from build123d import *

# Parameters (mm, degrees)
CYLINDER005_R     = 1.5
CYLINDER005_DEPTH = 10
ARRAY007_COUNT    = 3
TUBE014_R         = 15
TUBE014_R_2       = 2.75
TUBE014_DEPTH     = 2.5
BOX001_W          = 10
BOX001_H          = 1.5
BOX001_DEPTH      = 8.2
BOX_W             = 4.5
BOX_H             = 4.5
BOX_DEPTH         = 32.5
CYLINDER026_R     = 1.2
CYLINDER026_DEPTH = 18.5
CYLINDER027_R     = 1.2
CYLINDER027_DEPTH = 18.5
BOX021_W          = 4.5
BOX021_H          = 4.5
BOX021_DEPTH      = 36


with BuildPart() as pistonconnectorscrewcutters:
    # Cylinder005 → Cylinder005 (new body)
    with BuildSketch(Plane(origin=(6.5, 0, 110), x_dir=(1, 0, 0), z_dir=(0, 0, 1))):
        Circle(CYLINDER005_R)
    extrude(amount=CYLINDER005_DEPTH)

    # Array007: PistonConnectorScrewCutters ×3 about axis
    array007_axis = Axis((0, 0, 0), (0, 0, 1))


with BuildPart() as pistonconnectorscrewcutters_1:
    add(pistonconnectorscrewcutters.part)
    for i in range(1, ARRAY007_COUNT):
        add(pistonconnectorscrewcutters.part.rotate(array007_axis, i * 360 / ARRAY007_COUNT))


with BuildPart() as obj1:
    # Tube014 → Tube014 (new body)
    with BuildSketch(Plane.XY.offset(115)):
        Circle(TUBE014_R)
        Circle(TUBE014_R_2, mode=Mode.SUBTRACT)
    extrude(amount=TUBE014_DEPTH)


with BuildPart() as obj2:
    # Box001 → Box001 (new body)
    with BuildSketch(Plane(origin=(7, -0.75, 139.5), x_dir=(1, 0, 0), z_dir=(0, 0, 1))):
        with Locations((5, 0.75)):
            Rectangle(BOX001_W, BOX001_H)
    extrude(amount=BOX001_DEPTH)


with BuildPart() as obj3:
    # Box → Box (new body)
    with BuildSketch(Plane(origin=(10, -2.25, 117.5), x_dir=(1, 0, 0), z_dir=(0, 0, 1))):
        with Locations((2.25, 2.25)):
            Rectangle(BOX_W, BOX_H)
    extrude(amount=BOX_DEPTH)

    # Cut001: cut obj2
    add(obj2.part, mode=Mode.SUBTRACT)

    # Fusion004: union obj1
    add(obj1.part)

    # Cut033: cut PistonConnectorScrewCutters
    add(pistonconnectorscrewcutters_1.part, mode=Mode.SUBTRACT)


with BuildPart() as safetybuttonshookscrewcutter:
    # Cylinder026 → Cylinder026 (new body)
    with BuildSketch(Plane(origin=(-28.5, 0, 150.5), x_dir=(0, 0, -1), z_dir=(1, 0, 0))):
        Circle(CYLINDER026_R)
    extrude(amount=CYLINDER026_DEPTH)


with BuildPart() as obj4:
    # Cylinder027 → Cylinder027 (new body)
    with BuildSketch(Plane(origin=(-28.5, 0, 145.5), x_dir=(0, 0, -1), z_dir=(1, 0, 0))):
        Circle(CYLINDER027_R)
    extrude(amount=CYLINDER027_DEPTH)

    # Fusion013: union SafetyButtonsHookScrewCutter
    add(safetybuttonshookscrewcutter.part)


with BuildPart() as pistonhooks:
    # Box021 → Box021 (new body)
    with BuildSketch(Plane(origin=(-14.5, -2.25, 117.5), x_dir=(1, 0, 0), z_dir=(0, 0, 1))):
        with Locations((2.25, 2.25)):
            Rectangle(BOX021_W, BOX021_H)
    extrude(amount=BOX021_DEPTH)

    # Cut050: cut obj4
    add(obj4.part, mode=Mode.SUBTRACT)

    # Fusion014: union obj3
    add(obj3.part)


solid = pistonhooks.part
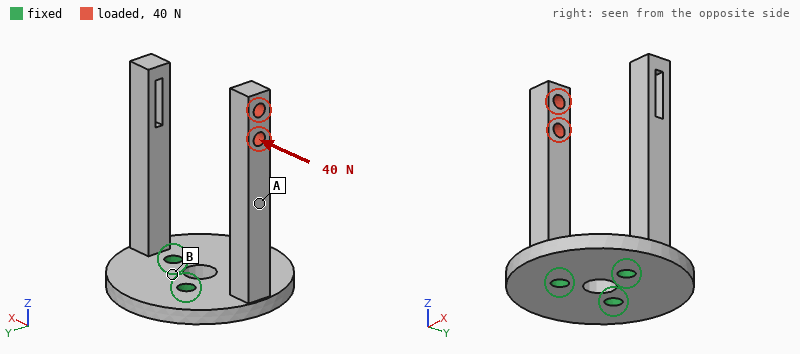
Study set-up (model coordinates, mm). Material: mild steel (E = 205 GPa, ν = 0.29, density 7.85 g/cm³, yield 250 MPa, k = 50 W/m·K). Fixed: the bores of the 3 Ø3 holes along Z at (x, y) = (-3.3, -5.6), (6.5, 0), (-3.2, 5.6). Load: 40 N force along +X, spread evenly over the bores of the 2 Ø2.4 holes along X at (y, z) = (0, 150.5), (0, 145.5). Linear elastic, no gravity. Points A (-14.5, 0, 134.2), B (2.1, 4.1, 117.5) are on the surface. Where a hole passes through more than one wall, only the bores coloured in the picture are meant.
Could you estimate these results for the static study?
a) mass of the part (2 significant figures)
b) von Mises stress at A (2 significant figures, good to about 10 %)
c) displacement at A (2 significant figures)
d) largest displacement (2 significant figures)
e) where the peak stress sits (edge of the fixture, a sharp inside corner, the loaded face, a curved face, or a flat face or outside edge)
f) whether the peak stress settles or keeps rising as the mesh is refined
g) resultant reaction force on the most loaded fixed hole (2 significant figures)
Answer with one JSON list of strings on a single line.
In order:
["23 g", "36 MPa", "0.061 mm", "0.15 mm", "edge of the fixture", "keeps rising", "25 N"]
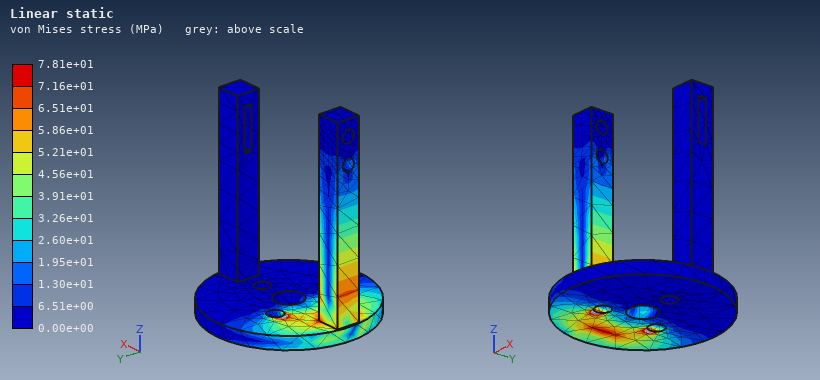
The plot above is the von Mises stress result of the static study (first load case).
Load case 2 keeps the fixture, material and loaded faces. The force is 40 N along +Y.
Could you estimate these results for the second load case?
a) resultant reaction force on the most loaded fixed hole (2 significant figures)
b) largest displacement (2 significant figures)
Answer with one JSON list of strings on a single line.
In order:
["120 N", "0.11 mm"]
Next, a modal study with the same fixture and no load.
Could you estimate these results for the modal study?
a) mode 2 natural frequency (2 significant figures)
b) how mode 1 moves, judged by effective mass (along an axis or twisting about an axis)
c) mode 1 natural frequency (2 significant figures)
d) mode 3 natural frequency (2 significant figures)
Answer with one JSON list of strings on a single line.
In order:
["2400 Hz", "along X", "1900 Hz", "2500 Hz"]
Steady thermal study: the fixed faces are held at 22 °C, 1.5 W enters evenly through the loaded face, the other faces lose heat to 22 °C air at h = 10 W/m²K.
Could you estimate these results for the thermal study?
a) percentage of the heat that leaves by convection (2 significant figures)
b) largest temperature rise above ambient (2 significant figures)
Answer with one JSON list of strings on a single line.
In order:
["14 %", "51 K"]
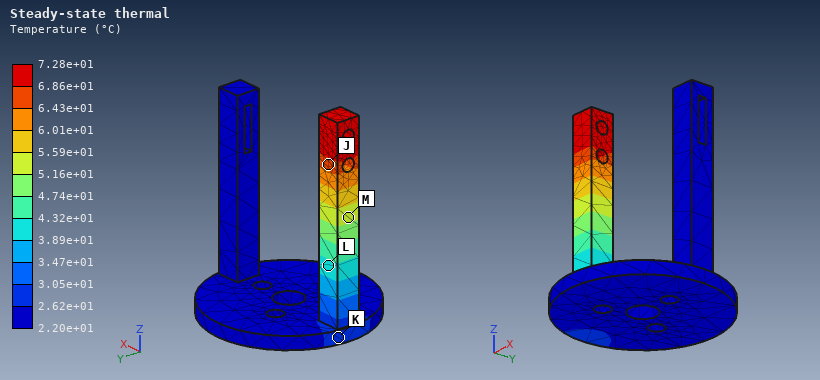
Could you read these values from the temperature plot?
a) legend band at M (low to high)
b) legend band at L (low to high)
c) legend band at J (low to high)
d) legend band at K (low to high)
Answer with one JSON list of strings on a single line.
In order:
["5.16e+01 to 5.59e+01 °C", "3.89e+01 to 4.32e+01 °C", "6.43e+01 to 6.86e+01 °C", "2.62e+01 to 3.05e+01 °C"]
